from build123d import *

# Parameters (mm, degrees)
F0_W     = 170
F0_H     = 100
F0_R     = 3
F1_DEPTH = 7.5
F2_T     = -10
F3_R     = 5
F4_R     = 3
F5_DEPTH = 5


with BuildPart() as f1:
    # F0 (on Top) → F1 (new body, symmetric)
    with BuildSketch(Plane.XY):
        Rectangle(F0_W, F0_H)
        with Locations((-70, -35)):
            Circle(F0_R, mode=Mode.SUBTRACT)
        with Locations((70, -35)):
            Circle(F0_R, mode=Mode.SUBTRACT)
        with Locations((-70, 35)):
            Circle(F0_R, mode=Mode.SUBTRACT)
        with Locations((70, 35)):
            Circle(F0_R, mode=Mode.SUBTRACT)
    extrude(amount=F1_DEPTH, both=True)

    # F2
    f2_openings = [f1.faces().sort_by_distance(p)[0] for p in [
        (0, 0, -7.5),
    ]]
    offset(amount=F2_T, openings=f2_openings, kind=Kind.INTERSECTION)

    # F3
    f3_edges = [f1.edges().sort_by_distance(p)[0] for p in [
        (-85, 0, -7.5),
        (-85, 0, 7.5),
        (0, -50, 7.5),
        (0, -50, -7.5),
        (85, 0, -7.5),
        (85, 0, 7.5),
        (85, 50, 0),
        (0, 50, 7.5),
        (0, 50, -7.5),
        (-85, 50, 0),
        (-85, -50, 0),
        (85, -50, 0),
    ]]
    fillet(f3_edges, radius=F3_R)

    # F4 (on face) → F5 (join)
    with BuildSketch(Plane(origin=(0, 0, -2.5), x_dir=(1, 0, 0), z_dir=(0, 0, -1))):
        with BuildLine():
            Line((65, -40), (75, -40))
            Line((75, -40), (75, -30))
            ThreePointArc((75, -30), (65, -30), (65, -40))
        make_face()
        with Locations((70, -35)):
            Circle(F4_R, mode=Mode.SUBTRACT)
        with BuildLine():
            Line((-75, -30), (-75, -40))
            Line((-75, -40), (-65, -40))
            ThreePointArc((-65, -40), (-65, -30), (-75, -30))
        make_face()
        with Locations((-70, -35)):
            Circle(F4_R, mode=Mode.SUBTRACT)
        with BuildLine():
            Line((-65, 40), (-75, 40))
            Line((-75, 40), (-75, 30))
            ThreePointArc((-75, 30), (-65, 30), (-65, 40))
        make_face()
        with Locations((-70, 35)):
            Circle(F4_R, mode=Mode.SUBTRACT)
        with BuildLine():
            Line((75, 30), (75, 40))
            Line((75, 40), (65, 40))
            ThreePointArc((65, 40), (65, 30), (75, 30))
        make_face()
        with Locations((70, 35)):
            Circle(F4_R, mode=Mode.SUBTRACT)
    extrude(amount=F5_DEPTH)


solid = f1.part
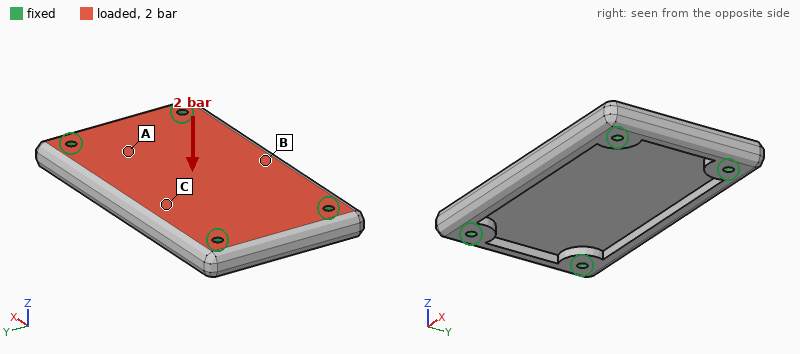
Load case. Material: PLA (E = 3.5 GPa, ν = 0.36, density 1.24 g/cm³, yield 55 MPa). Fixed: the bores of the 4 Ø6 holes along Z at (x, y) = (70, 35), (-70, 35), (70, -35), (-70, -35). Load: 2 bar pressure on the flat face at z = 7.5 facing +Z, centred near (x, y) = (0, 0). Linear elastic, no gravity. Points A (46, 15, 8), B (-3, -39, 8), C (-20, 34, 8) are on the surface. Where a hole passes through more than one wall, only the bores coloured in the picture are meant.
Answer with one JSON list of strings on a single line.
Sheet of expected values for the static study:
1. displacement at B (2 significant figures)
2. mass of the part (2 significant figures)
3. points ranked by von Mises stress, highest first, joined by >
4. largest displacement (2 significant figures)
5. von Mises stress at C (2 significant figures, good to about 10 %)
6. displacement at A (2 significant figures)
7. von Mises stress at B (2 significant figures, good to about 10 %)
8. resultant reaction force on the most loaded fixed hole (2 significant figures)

["0.43 mm", "240 g", "B > C > A", "0.51 mm", "5.2 MPa", "0.22 mm", "6.9 MPa", "750 N"]
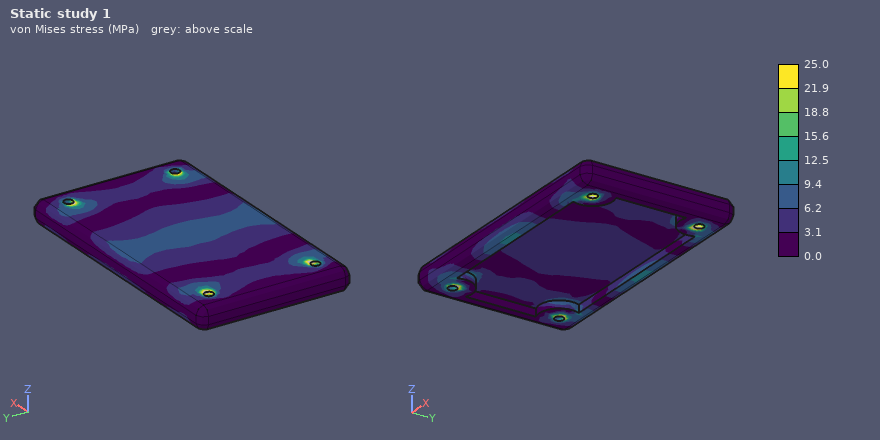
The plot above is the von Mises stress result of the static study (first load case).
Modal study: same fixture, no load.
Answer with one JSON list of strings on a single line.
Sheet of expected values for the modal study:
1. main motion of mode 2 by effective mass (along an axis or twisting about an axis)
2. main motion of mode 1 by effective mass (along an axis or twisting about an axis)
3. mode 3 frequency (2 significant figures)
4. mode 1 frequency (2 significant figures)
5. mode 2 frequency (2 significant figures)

["twisting about X", "along Z", "2300 Hz", "970 Hz", "1300 Hz"]
